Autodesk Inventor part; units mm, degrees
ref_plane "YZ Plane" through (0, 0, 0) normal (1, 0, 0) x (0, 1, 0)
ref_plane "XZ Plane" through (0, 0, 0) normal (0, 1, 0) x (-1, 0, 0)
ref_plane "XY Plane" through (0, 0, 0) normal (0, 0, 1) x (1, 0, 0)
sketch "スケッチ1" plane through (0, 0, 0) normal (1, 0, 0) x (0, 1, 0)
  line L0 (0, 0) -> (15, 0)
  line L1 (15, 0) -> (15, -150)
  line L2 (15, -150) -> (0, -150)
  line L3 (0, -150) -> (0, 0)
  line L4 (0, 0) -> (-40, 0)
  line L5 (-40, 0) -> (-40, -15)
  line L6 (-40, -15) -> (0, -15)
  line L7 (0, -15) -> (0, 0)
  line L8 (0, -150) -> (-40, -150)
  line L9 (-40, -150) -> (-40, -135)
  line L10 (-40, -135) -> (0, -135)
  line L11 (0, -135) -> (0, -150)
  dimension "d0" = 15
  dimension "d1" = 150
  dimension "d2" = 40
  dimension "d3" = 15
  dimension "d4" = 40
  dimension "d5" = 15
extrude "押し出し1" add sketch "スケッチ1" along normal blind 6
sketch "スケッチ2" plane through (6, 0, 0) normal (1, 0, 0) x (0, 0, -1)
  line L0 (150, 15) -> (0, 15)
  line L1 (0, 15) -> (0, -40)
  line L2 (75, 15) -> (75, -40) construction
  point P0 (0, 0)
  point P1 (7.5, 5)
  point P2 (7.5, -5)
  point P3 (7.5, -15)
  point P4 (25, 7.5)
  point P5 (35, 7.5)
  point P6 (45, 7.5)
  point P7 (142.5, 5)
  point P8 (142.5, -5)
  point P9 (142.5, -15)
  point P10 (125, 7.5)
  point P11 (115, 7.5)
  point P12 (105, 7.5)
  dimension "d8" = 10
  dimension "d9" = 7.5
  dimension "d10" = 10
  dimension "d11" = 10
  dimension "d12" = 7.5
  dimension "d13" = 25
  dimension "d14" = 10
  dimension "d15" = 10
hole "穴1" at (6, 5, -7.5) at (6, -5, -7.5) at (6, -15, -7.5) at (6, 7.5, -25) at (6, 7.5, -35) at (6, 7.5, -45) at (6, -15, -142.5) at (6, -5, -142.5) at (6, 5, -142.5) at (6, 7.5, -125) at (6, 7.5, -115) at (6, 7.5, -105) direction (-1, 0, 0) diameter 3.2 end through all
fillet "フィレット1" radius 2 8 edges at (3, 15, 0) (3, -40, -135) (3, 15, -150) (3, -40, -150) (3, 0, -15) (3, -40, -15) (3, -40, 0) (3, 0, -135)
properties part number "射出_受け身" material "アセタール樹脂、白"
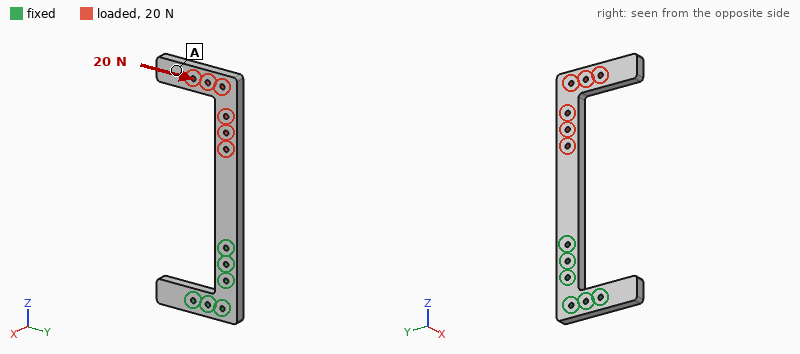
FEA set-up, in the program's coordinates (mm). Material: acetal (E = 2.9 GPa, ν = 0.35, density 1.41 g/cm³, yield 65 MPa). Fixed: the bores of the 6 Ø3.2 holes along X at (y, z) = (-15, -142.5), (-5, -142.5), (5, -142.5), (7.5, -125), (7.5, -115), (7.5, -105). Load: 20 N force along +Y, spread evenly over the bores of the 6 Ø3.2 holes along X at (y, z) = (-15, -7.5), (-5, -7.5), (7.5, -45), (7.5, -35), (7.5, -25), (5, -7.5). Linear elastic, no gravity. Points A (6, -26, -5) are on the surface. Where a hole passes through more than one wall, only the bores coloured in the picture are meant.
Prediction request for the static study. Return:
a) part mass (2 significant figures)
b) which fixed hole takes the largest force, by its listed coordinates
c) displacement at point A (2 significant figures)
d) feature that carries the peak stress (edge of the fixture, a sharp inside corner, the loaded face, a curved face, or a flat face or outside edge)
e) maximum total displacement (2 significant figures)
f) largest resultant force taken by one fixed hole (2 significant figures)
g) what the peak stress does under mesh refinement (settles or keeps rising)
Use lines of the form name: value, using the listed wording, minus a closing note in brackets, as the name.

part mass: 28 g
which fixed hole takes the largest force, by its listed coordinates: (7.5, -105)
displacement at point A: 1.4 mm
feature that carries the peak stress: edge of the fixture
maximum total displacement: 1.6 mm
largest resultant force taken by one fixed hole: 110 N
what the peak stress does under mesh refinement: keeps rising
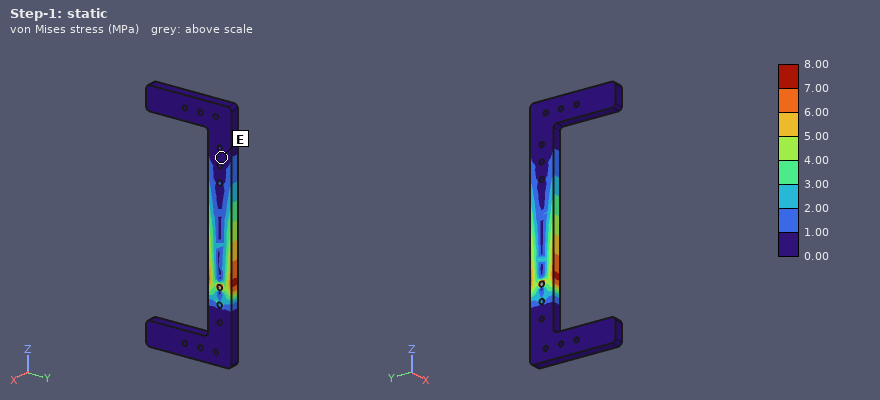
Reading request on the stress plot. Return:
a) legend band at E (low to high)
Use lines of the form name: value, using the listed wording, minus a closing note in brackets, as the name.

legend band at E: 0.00 to 1.00 MPa
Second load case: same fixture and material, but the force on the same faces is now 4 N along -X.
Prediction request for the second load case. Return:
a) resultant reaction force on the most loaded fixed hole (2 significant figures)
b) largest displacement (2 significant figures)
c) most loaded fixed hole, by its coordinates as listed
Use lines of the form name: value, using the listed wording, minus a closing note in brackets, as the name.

resultant reaction force on the most loaded fixed hole: 14 N
largest displacement: 1.6 mm
most loaded fixed hole, by its coordinates as listed: (7.5, -105)
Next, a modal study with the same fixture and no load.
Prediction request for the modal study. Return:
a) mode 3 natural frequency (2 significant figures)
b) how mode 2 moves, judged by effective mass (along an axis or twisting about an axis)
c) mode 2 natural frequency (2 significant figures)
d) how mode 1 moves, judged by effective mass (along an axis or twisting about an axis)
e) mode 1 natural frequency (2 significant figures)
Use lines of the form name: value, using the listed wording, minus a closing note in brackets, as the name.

mode 3 natural frequency: 290 Hz
how mode 2 moves, judged by effective mass: along Y
mode 2 natural frequency: 180 Hz
how mode 1 moves, judged by effective mass: along X
mode 1 natural frequency: 81 Hz
